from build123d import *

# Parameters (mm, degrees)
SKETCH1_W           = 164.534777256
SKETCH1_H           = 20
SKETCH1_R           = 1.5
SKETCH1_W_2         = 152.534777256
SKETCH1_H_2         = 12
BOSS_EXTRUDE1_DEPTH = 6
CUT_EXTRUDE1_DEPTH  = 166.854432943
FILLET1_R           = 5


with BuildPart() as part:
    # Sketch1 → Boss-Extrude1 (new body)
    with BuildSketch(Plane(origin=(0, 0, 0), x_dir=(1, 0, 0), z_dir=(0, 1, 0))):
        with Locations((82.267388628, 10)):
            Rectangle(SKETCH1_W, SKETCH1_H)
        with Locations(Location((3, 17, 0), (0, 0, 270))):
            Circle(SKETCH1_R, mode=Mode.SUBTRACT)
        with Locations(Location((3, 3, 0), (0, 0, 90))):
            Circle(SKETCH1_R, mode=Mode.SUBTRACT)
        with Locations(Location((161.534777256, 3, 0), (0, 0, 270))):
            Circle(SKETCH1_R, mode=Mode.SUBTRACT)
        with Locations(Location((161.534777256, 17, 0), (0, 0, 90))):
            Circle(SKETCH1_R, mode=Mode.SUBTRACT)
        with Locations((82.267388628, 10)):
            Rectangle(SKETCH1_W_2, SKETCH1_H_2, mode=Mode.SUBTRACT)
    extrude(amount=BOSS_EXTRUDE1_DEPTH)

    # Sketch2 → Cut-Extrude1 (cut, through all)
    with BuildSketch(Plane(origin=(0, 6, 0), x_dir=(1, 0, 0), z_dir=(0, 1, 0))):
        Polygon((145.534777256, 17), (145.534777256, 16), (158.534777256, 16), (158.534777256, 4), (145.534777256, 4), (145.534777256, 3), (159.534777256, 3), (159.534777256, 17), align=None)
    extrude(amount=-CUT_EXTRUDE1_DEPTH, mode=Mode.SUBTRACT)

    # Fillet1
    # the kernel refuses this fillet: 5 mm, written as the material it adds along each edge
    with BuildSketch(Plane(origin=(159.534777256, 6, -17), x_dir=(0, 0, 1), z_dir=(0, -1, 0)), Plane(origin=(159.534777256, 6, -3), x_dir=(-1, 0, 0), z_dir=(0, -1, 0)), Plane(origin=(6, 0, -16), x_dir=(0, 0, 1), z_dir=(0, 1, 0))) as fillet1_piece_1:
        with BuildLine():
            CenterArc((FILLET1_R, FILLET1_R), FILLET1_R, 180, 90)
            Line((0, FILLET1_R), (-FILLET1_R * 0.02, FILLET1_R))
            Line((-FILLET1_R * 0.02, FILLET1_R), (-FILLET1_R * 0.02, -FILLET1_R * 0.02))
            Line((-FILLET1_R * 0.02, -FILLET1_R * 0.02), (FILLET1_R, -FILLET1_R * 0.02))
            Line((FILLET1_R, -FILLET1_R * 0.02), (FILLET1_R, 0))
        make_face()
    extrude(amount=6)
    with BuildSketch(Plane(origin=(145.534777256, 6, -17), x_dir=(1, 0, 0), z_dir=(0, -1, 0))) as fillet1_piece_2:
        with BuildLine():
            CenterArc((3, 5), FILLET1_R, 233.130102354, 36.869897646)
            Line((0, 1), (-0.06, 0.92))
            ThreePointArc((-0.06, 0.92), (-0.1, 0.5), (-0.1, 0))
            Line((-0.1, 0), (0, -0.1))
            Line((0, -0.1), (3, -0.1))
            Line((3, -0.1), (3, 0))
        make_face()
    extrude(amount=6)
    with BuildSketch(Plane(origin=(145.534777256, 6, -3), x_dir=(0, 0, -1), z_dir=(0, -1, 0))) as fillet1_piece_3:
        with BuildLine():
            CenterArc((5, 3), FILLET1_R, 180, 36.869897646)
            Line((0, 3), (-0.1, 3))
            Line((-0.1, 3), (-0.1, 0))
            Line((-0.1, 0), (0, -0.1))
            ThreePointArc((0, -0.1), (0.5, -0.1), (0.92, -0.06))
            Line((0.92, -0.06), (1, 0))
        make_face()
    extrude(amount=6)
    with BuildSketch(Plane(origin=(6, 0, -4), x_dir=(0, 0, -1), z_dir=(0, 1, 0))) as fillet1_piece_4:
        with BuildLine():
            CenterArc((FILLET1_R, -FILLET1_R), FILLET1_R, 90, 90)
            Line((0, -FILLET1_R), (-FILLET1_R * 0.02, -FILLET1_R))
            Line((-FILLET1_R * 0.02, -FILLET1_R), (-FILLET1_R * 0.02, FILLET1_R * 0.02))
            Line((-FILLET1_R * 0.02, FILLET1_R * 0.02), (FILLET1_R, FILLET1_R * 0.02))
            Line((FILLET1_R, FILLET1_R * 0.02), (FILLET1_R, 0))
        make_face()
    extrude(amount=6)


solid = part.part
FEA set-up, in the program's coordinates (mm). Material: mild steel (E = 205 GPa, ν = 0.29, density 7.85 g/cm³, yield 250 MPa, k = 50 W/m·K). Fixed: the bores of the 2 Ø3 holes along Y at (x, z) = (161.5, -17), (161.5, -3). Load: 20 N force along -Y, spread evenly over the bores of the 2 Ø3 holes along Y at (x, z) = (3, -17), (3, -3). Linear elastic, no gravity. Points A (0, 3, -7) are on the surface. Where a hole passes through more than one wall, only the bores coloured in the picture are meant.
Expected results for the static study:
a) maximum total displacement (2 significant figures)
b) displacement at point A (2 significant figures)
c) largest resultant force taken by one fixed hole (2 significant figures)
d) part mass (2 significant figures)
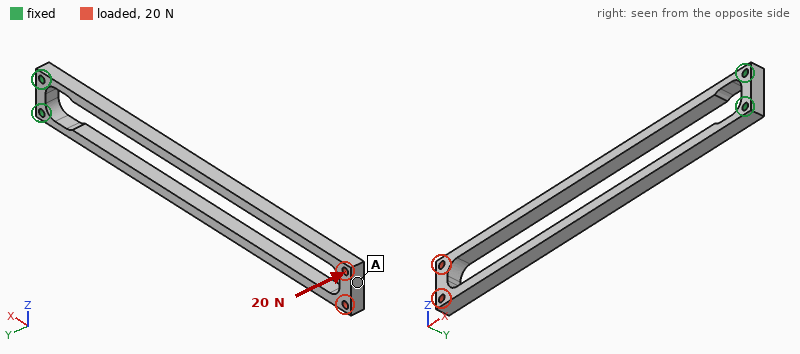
0.97 mm
0.97 mm
10 N
67 g
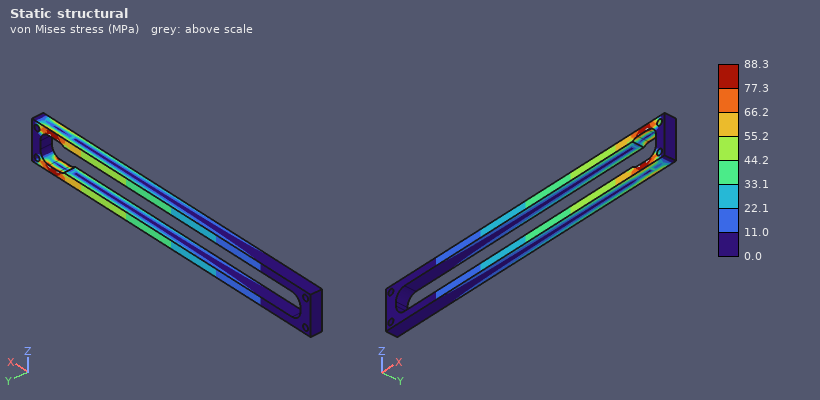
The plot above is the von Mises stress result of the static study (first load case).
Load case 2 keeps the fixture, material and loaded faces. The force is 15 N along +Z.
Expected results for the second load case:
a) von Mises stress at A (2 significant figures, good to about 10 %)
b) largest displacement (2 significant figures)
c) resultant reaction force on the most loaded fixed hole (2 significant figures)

5.5 MPa
0.42 mm
100 N
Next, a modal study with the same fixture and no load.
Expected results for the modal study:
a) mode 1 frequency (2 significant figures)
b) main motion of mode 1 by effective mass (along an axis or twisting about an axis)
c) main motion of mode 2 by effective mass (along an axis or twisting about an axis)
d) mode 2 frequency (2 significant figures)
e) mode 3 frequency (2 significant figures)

170 Hz
along Y
along Z
180 Hz
800 Hz
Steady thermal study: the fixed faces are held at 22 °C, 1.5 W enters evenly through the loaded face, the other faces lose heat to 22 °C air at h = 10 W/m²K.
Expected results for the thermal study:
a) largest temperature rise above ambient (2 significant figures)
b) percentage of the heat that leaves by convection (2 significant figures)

42 K
77 %
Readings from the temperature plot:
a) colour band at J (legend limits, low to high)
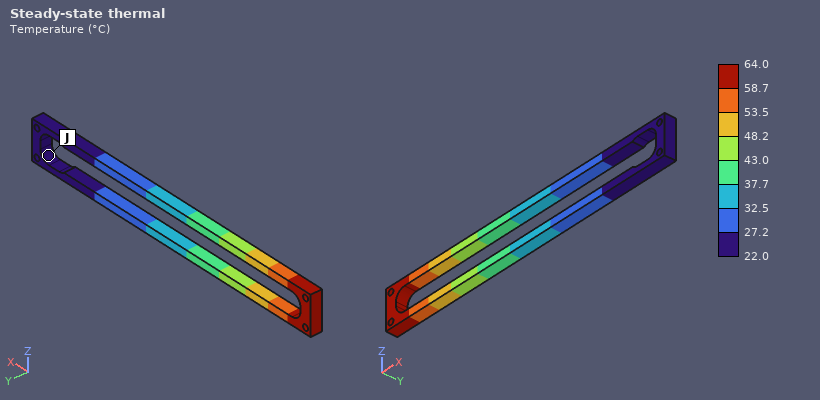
22.0 to 27.2 °C
